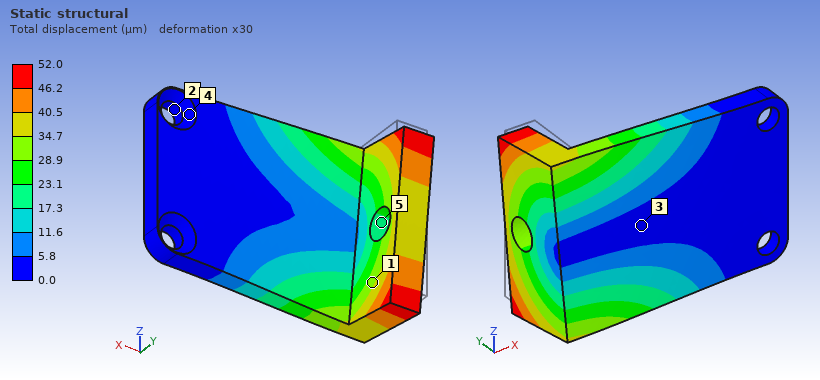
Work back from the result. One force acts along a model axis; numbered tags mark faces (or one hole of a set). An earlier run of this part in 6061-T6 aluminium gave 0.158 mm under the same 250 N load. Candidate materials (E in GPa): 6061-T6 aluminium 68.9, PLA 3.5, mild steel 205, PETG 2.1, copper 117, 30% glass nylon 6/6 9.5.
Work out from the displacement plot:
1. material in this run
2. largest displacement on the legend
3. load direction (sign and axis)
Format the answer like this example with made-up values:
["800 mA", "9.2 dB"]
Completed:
["mild steel", "52.0 µm", "-Z"]
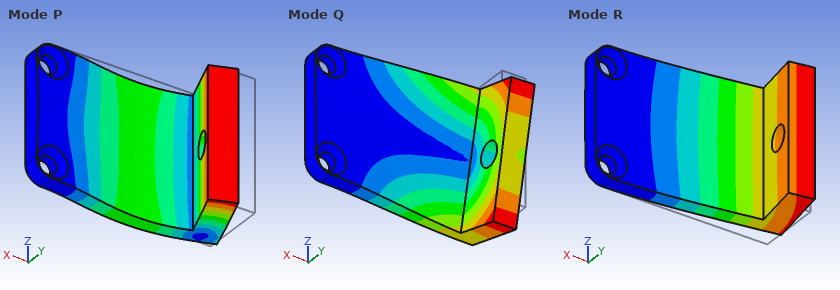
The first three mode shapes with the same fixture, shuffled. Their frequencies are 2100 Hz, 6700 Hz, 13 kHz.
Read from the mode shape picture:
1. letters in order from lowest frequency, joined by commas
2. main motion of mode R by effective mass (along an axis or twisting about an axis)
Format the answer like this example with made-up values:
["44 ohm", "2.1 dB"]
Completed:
["R, Q, P", "along Y"]
